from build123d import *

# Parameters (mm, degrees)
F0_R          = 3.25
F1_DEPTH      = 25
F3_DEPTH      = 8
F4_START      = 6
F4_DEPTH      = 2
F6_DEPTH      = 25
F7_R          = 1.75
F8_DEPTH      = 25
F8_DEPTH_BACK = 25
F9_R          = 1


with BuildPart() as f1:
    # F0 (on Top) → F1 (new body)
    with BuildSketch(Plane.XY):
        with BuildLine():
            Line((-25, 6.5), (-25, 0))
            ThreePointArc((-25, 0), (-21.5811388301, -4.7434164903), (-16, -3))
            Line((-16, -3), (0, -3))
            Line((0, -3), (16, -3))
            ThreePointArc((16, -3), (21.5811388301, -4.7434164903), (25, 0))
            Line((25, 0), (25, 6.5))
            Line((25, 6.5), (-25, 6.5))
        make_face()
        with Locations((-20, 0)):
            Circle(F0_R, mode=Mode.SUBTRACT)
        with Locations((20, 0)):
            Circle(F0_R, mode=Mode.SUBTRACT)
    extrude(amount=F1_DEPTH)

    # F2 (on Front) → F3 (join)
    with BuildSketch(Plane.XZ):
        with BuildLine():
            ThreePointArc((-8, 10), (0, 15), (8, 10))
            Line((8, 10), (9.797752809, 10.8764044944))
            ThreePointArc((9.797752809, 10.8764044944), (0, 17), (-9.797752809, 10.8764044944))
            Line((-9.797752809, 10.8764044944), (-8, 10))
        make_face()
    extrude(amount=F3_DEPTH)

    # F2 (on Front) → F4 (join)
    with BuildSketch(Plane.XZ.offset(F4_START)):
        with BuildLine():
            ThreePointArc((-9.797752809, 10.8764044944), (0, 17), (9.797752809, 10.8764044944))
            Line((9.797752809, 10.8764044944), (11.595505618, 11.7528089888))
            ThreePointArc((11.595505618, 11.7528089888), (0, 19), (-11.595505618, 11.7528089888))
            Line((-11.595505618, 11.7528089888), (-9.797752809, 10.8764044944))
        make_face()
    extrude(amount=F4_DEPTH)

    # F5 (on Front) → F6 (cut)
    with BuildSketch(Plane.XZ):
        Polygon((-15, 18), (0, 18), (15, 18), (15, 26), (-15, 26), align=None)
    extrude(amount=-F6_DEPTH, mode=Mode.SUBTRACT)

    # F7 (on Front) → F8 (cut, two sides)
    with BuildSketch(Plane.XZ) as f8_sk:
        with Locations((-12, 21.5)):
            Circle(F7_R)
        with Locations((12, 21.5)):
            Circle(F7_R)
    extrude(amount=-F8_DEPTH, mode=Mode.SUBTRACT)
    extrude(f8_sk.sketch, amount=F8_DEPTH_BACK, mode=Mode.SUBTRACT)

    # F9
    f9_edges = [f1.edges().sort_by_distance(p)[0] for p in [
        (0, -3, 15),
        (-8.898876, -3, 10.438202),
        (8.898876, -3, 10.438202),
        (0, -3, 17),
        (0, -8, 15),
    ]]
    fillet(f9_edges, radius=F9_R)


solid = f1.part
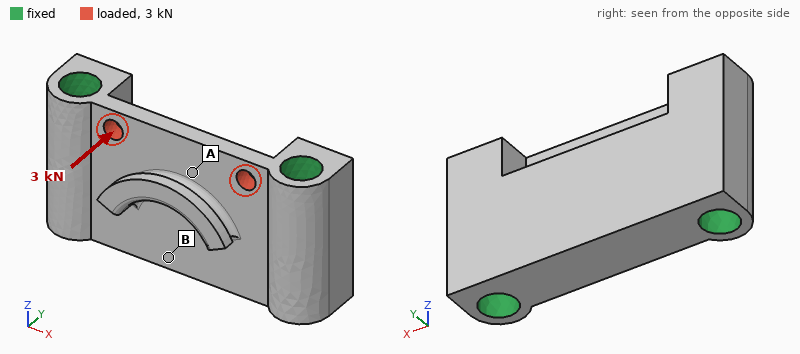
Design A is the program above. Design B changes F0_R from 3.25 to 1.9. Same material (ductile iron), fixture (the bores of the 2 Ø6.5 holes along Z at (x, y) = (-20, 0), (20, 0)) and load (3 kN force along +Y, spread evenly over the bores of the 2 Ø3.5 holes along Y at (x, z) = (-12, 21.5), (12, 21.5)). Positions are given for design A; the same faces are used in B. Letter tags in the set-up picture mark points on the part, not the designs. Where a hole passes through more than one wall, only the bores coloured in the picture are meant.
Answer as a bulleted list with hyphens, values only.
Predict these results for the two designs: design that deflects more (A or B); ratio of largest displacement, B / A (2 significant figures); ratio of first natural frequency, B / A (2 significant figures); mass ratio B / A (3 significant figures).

- B
- 1.1
- 0.88
- 1.11
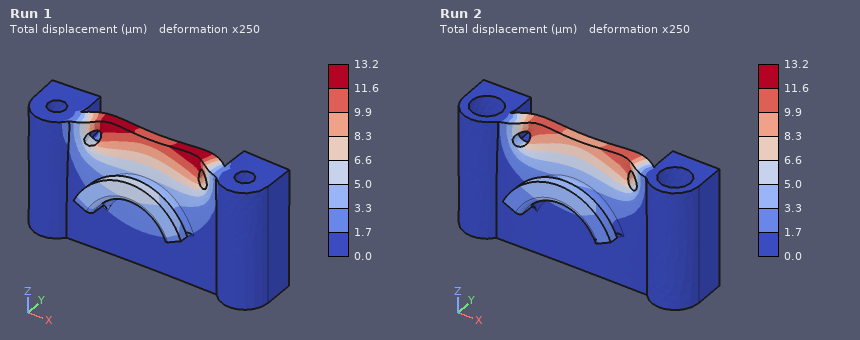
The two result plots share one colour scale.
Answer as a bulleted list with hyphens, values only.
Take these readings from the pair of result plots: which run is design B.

- Run 1
